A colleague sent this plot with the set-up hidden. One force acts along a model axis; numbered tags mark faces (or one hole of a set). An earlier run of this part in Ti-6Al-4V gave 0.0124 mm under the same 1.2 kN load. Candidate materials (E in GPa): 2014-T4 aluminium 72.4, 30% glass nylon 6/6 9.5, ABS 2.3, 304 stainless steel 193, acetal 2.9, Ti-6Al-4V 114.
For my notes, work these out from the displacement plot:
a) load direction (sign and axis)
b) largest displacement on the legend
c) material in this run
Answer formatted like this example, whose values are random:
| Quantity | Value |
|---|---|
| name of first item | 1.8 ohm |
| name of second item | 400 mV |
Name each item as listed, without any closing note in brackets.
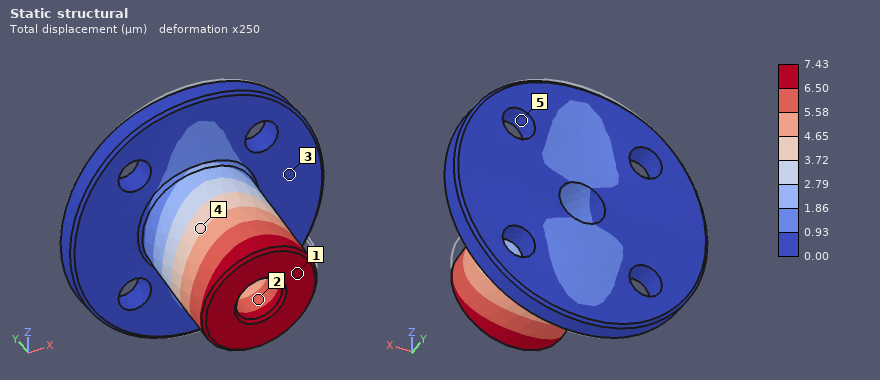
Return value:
| Quantity | Value |
|---|---|
| load direction | -Z |
| largest displacement on the legend | 7.43 µm |
| material in this run | 304 stainless steel |
